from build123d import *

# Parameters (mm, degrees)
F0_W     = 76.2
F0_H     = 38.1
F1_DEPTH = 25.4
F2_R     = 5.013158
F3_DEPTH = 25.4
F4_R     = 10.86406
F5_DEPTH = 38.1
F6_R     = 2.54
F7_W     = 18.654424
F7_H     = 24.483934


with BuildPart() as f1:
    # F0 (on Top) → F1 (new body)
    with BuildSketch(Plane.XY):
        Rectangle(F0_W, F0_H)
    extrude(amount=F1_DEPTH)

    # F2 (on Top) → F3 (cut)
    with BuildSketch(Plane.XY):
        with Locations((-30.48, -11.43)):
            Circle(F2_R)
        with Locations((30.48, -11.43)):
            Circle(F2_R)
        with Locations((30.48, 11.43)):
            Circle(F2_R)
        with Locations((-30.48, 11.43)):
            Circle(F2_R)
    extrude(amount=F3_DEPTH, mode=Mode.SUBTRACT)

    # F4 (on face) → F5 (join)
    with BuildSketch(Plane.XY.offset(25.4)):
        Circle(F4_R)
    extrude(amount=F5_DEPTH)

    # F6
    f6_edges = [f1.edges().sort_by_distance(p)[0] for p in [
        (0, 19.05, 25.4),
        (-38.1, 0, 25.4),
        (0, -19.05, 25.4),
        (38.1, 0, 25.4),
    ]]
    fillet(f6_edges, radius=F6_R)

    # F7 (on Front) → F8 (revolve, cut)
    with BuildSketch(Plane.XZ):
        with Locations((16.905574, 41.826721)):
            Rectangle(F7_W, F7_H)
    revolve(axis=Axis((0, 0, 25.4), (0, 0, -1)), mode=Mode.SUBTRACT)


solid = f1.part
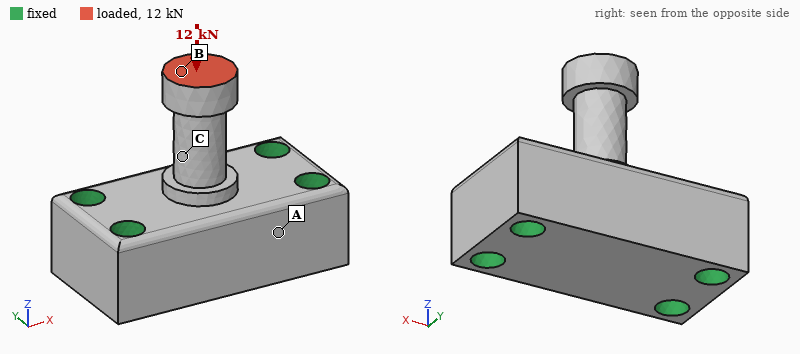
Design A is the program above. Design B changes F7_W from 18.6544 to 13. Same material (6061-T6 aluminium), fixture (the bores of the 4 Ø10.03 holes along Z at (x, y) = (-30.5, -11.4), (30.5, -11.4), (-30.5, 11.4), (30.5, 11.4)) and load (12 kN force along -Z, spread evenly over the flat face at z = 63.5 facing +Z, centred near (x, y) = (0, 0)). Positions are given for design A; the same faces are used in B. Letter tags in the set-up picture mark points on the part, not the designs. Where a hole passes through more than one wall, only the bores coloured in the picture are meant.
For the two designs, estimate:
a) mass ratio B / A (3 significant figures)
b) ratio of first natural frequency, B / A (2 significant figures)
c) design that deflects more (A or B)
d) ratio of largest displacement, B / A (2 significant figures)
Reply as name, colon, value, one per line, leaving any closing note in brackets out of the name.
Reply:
mass ratio B / A: 1.05
ratio of first natural frequency, B / A: 1.3
design that deflects more: A
ratio of largest displacement, B / A: 0.67
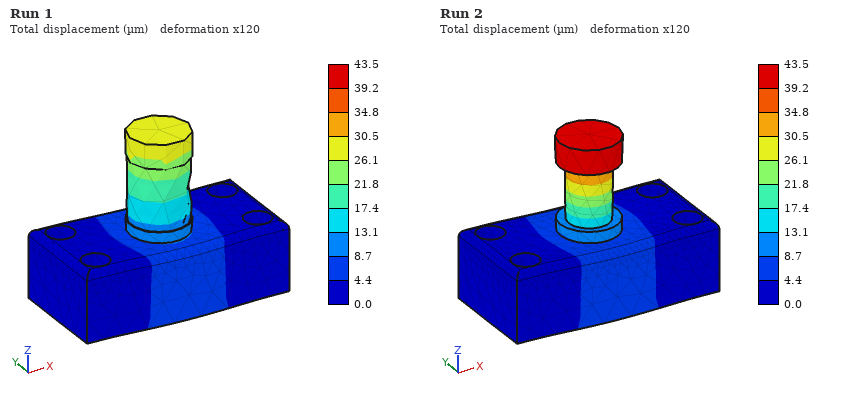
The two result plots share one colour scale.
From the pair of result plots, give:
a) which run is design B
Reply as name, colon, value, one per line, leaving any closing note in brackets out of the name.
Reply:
which run is design B: Run 1
